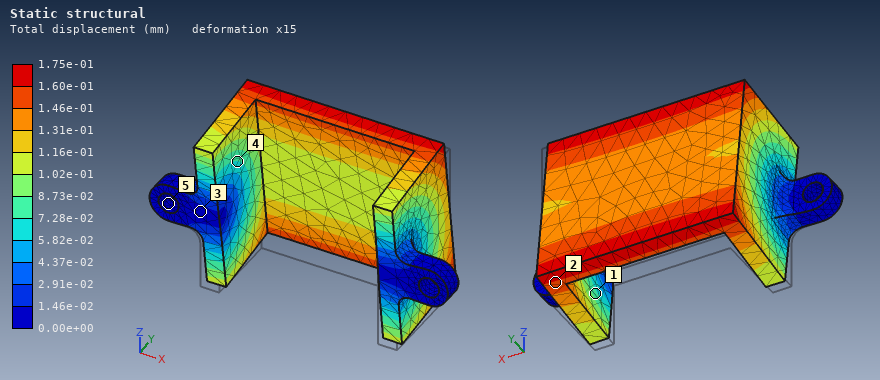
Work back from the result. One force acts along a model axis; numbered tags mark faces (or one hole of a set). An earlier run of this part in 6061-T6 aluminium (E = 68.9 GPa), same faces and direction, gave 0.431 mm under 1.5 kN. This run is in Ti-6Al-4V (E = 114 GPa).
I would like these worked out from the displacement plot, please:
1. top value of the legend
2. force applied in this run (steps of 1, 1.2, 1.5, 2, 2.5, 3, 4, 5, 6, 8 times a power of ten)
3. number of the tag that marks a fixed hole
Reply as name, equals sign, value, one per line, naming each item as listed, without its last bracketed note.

top value of the legend = 1.75e-01 mm
force applied in this run = 1 kN
number of the tag that marks a fixed hole = 5
